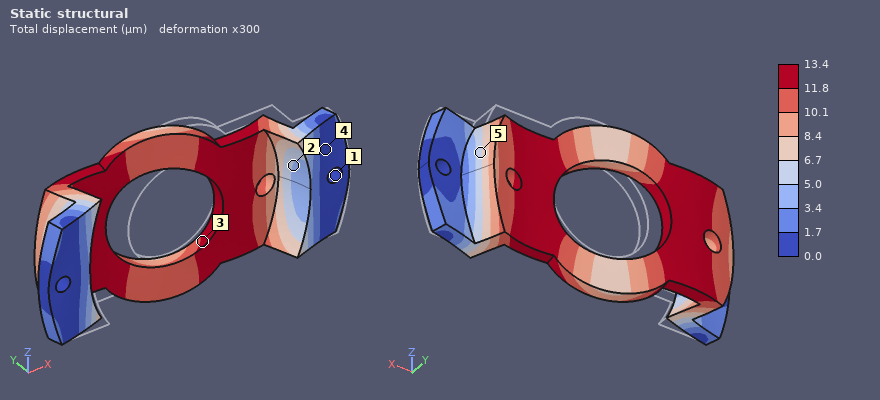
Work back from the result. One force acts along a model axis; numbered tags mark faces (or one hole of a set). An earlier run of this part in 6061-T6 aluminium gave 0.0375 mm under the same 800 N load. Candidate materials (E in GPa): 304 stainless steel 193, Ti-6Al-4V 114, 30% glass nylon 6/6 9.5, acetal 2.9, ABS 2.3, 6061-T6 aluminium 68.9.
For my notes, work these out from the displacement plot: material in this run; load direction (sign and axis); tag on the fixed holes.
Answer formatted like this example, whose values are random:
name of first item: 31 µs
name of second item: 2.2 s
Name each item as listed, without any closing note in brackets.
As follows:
material in this run: 304 stainless steel
load direction: -X
tag on the fixed holes: 1
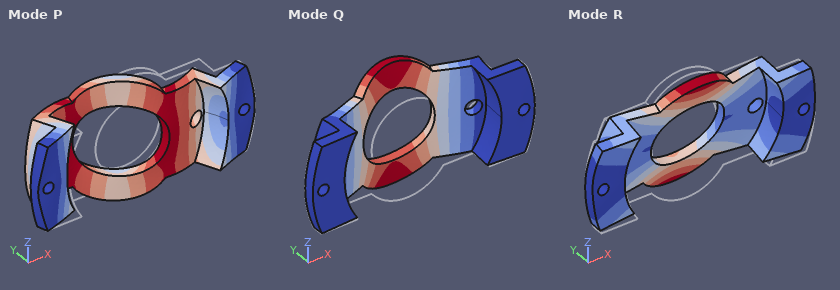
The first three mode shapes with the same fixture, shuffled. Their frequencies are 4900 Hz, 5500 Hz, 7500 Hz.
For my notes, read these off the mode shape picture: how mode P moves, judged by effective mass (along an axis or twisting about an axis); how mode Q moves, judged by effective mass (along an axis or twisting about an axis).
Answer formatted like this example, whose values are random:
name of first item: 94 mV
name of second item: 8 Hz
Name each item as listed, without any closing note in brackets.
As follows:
how mode P moves, judged by effective mass: along X
how mode Q moves, judged by effective mass: along Y
